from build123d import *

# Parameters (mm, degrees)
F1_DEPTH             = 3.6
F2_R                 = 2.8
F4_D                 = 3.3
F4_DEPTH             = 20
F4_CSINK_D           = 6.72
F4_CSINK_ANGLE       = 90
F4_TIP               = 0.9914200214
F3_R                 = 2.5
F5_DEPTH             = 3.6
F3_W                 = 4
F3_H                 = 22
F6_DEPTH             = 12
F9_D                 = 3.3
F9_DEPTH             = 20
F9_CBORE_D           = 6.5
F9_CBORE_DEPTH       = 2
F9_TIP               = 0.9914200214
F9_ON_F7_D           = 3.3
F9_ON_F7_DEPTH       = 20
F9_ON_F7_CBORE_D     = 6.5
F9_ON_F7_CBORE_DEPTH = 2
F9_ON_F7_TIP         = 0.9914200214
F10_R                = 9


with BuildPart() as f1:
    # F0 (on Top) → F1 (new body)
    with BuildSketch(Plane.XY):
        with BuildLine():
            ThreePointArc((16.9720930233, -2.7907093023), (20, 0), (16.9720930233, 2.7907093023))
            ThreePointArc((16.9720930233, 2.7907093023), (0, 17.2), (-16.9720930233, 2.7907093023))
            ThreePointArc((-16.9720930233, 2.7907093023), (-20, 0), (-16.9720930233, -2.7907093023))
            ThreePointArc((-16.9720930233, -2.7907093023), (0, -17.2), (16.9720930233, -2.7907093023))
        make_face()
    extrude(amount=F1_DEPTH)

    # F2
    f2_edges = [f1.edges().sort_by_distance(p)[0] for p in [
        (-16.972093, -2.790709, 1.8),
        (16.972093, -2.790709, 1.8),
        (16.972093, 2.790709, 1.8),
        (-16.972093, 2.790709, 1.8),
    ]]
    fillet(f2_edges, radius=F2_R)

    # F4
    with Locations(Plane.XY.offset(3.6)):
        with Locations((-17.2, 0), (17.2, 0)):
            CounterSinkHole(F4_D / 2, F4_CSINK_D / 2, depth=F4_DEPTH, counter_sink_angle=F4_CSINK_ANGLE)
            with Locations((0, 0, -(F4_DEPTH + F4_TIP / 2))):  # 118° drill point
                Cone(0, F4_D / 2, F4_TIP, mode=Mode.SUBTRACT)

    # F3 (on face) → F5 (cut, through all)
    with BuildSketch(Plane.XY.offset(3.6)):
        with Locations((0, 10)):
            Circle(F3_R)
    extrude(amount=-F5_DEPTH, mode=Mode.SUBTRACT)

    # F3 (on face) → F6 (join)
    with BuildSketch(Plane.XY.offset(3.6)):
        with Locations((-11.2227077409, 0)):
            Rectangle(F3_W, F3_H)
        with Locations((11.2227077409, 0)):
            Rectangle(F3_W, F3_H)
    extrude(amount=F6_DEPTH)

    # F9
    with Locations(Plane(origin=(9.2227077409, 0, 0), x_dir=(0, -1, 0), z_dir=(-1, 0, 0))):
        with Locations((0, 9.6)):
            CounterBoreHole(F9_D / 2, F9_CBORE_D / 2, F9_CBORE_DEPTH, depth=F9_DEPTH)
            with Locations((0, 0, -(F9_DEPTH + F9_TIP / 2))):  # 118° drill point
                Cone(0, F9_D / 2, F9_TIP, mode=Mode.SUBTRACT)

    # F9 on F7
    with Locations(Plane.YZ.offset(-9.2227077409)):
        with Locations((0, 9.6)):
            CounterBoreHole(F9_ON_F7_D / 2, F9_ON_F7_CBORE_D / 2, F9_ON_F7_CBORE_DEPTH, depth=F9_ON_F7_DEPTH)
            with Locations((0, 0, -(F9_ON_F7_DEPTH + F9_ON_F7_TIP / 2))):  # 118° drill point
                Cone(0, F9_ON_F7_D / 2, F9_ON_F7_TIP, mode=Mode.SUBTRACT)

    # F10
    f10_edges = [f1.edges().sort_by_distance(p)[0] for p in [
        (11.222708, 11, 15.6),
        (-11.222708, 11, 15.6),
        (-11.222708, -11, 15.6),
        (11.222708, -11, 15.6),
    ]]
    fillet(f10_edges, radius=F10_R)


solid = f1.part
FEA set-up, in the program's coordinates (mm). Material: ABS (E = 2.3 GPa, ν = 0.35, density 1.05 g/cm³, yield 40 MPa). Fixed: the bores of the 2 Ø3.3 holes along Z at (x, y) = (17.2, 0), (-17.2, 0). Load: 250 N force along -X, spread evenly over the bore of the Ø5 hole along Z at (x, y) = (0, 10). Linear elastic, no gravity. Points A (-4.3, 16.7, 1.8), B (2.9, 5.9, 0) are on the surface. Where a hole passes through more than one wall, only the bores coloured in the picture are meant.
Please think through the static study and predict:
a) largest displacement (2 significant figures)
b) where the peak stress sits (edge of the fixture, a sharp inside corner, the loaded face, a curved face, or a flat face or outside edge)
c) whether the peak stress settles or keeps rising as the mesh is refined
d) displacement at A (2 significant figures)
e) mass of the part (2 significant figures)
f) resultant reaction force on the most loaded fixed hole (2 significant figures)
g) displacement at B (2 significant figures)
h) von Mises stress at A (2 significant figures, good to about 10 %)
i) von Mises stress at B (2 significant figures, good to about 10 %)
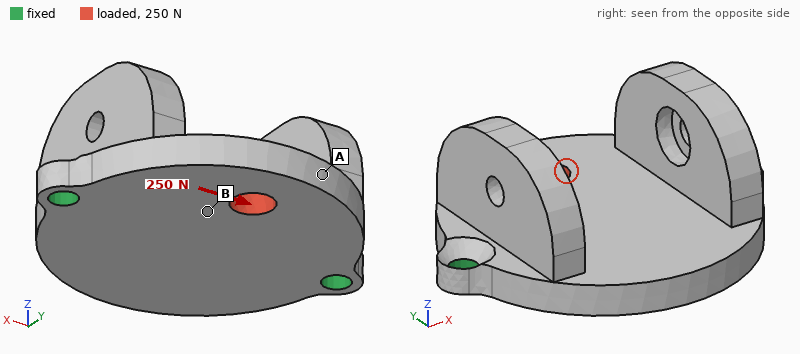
60 µm
edge of the fixture
keeps rising
50 µm
5.2 g
140 N
33 µm
1.7 MPa
4.5 MPa
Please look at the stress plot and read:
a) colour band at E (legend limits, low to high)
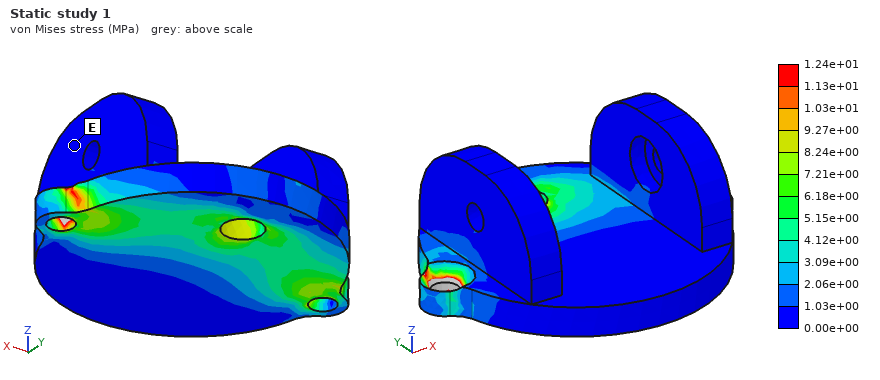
0.00e+00 to 1.03e+00 MPa
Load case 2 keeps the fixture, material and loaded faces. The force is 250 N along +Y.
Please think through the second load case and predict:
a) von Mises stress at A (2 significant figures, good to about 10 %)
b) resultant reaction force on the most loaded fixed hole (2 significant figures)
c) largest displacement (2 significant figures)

4.0 MPa
130 N
0.10 mm
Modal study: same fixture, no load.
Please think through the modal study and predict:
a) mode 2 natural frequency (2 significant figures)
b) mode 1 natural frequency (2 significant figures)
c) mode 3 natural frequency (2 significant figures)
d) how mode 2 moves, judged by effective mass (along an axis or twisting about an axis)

2200 Hz
1300 Hz
3500 Hz
along Z
